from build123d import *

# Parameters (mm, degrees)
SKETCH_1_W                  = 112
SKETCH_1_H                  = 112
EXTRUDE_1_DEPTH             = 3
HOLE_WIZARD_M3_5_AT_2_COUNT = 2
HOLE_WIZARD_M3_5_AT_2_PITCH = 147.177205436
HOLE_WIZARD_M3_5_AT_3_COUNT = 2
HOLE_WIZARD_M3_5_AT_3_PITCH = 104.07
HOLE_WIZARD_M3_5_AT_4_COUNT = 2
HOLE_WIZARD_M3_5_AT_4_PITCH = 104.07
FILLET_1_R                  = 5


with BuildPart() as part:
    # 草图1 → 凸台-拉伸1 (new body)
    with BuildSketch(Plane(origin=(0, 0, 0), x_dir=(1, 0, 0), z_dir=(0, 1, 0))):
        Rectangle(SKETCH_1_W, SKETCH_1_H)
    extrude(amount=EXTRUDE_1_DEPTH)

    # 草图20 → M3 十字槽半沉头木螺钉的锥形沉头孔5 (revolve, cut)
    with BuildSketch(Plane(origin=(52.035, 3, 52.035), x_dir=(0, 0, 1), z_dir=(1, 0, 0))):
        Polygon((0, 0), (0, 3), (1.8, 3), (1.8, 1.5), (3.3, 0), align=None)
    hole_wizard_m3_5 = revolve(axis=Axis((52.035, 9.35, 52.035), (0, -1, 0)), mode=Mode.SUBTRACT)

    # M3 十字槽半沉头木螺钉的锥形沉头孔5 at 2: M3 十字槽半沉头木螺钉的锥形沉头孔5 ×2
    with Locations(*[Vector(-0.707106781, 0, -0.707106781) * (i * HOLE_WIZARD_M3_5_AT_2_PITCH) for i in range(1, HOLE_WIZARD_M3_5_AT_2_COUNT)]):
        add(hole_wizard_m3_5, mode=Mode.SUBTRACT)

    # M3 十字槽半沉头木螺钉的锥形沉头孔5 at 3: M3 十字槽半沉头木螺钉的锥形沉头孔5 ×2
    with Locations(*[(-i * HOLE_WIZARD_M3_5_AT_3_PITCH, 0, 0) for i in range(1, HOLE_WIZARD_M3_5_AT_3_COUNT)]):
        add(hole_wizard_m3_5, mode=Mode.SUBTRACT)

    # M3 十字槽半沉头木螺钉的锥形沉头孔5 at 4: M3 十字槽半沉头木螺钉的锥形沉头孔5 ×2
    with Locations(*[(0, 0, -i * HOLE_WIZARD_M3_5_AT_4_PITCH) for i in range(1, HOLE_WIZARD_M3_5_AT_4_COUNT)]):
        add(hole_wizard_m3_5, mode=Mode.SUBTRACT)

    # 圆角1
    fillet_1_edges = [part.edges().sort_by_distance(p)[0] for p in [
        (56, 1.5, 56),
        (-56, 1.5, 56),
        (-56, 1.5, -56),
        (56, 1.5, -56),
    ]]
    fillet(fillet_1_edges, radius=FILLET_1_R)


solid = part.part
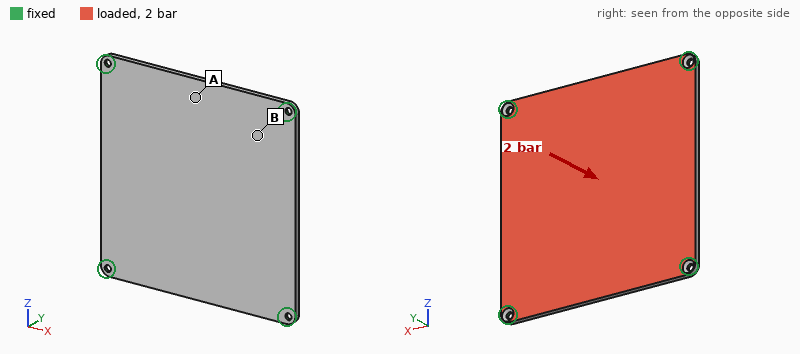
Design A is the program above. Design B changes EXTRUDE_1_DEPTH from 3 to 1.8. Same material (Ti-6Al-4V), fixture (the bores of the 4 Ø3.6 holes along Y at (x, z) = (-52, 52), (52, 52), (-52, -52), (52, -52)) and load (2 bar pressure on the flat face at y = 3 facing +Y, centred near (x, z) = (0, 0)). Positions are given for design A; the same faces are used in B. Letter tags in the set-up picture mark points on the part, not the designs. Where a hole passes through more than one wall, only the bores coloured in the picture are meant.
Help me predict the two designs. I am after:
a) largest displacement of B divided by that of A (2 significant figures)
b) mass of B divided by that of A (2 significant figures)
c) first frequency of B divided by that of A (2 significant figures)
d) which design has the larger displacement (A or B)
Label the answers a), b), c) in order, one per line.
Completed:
a) 3.8
b) 0.60
c) 0.67
d) B
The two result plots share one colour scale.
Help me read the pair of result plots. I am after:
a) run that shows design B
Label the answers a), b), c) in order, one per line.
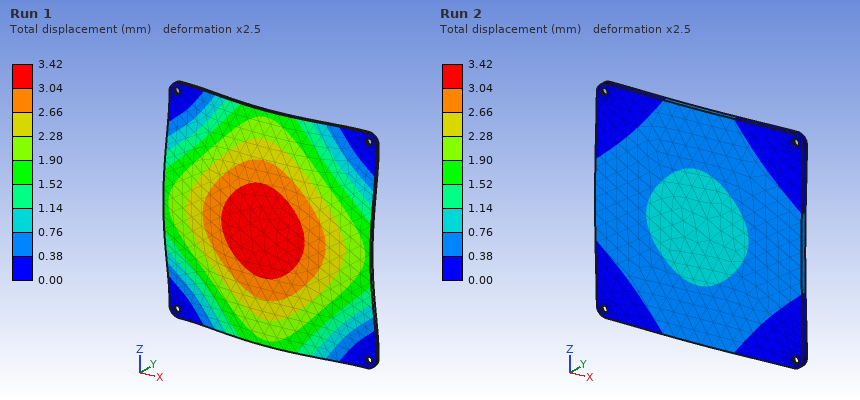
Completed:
a) Run 1
